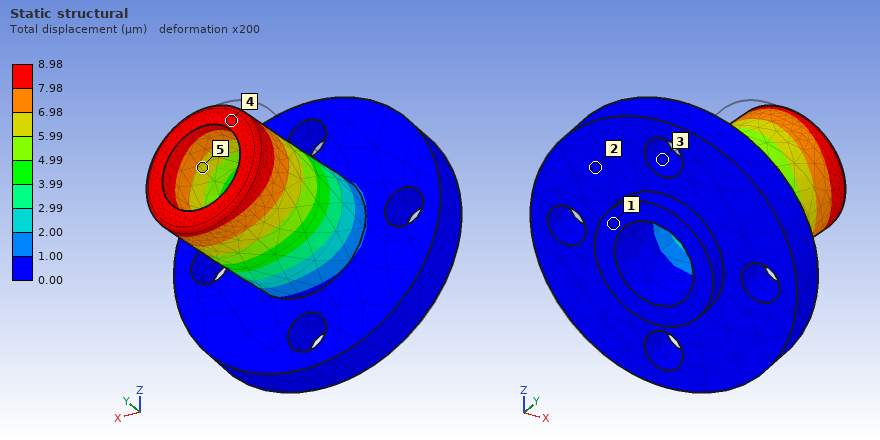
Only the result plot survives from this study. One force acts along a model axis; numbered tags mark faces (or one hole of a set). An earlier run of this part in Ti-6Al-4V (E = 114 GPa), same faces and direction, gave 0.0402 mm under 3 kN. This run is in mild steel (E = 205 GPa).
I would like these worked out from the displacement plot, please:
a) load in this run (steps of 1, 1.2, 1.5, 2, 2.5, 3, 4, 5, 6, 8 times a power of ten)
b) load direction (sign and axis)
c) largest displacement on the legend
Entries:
1.2 kN
+X
8.98 µm
